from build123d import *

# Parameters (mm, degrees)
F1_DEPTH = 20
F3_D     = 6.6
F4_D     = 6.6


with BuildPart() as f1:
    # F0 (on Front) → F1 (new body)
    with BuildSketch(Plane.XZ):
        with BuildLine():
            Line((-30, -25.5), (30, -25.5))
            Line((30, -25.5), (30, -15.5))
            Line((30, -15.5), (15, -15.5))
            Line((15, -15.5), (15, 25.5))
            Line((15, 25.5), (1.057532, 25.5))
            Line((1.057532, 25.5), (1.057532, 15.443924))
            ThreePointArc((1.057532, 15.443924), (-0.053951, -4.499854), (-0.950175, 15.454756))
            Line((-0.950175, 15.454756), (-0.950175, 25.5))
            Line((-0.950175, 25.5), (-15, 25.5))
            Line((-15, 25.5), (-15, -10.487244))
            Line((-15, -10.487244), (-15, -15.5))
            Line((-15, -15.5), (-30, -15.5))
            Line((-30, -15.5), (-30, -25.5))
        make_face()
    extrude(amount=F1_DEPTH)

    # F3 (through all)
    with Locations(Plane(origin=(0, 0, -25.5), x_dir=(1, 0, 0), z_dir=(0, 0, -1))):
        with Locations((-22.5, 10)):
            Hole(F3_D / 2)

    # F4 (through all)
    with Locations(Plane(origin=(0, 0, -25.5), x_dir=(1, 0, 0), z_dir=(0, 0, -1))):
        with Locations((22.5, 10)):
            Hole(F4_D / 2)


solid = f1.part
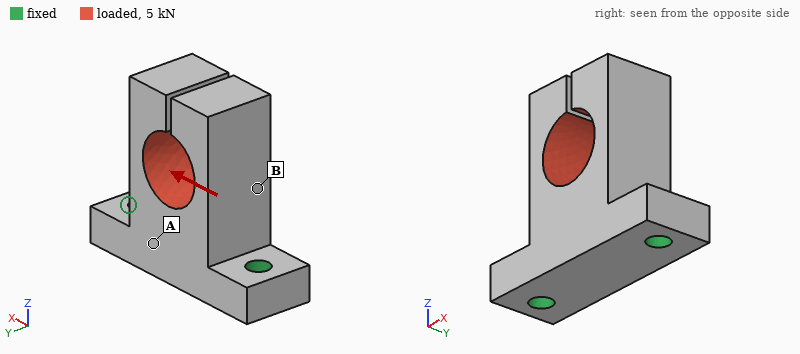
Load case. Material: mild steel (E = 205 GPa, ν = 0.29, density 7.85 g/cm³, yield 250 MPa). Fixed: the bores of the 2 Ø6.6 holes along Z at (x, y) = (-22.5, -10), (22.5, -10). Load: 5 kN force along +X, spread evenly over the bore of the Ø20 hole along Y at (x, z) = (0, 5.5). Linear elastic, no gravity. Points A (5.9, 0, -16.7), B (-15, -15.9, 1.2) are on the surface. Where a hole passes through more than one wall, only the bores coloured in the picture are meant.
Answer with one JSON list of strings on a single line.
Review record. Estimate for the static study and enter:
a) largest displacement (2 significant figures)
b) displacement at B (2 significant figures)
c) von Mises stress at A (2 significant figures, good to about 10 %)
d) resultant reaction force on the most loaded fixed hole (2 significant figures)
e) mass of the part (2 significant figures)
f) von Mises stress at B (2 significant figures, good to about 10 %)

["81 µm", "15 µm", "16 MPa", "4.3 kN", "230 g", "110 MPa"]
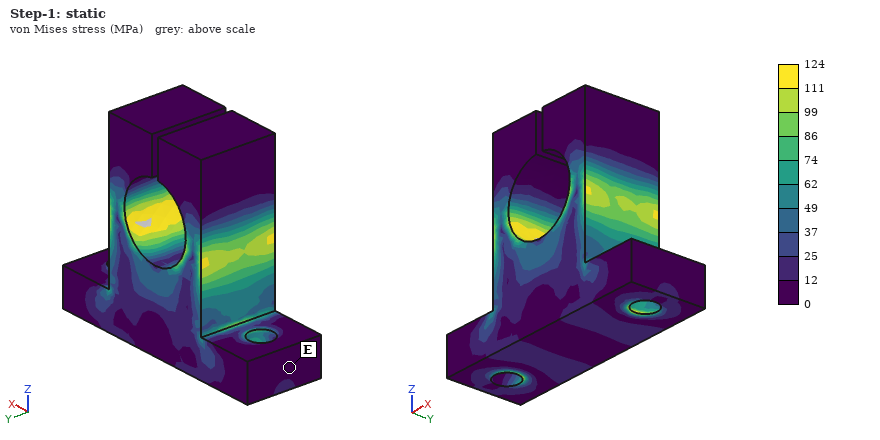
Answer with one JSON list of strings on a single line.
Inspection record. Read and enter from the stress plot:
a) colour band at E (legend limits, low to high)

["0 to 12 MPa"]
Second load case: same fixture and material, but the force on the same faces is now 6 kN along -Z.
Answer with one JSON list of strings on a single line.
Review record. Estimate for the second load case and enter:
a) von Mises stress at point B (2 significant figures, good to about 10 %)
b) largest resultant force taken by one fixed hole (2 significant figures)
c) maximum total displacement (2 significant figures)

["57 MPa", "3.2 kN", "56 µm"]
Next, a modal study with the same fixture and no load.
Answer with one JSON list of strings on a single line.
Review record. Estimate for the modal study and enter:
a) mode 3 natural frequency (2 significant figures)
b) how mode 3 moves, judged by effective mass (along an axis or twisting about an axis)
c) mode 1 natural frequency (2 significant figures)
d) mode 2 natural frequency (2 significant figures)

["3600 Hz", "along Y", "3300 Hz", "3400 Hz"]
